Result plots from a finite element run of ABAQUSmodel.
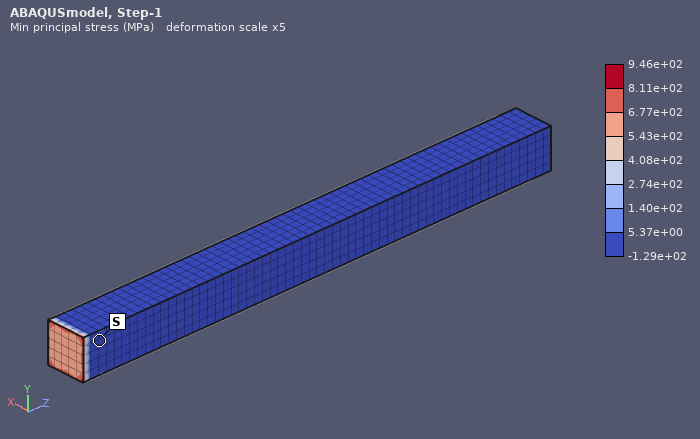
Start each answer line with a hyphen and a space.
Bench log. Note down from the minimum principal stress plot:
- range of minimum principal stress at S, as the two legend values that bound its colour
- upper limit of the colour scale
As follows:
- -1.29e+02 to 5.37e+00 MPa
- 9.46e+02 MPa
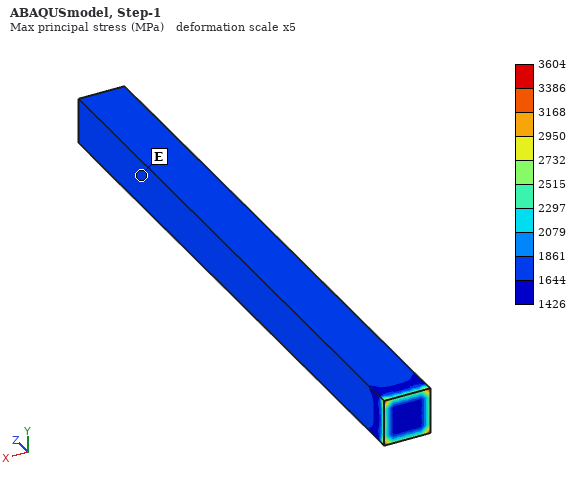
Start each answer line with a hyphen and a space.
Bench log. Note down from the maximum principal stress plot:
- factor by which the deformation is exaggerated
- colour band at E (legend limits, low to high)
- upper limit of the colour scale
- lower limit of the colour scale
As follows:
- 5
- 1644 to 1861 MPa
- 3604 MPa
- 1426 MPa
